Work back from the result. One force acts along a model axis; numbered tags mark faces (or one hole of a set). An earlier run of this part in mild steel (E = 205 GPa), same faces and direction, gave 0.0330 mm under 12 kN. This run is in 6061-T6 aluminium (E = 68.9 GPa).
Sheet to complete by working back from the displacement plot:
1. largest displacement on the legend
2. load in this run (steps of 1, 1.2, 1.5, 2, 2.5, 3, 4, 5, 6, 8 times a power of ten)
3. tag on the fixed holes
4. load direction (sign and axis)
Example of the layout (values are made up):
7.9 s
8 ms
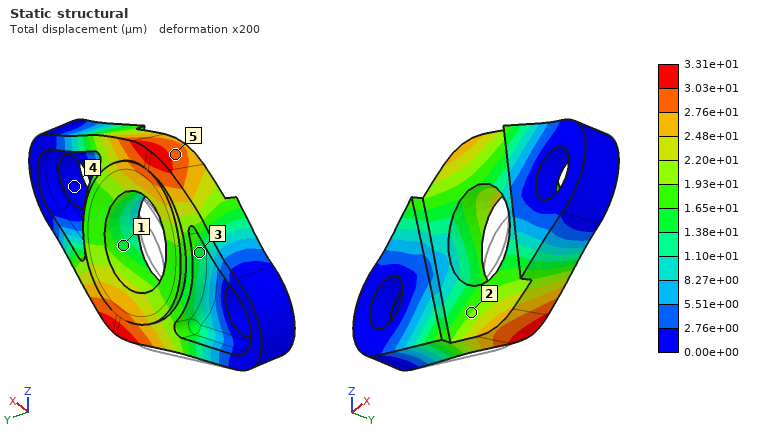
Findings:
3.31e+01 µm
4 kN
4
+Z
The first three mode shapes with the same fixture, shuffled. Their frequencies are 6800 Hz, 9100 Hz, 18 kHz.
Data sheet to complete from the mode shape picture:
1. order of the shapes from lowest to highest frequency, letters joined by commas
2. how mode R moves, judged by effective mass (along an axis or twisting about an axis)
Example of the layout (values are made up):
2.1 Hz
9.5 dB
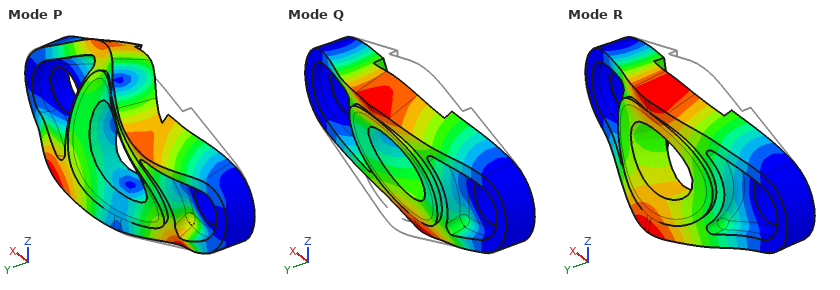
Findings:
Q, R, P
along Y
